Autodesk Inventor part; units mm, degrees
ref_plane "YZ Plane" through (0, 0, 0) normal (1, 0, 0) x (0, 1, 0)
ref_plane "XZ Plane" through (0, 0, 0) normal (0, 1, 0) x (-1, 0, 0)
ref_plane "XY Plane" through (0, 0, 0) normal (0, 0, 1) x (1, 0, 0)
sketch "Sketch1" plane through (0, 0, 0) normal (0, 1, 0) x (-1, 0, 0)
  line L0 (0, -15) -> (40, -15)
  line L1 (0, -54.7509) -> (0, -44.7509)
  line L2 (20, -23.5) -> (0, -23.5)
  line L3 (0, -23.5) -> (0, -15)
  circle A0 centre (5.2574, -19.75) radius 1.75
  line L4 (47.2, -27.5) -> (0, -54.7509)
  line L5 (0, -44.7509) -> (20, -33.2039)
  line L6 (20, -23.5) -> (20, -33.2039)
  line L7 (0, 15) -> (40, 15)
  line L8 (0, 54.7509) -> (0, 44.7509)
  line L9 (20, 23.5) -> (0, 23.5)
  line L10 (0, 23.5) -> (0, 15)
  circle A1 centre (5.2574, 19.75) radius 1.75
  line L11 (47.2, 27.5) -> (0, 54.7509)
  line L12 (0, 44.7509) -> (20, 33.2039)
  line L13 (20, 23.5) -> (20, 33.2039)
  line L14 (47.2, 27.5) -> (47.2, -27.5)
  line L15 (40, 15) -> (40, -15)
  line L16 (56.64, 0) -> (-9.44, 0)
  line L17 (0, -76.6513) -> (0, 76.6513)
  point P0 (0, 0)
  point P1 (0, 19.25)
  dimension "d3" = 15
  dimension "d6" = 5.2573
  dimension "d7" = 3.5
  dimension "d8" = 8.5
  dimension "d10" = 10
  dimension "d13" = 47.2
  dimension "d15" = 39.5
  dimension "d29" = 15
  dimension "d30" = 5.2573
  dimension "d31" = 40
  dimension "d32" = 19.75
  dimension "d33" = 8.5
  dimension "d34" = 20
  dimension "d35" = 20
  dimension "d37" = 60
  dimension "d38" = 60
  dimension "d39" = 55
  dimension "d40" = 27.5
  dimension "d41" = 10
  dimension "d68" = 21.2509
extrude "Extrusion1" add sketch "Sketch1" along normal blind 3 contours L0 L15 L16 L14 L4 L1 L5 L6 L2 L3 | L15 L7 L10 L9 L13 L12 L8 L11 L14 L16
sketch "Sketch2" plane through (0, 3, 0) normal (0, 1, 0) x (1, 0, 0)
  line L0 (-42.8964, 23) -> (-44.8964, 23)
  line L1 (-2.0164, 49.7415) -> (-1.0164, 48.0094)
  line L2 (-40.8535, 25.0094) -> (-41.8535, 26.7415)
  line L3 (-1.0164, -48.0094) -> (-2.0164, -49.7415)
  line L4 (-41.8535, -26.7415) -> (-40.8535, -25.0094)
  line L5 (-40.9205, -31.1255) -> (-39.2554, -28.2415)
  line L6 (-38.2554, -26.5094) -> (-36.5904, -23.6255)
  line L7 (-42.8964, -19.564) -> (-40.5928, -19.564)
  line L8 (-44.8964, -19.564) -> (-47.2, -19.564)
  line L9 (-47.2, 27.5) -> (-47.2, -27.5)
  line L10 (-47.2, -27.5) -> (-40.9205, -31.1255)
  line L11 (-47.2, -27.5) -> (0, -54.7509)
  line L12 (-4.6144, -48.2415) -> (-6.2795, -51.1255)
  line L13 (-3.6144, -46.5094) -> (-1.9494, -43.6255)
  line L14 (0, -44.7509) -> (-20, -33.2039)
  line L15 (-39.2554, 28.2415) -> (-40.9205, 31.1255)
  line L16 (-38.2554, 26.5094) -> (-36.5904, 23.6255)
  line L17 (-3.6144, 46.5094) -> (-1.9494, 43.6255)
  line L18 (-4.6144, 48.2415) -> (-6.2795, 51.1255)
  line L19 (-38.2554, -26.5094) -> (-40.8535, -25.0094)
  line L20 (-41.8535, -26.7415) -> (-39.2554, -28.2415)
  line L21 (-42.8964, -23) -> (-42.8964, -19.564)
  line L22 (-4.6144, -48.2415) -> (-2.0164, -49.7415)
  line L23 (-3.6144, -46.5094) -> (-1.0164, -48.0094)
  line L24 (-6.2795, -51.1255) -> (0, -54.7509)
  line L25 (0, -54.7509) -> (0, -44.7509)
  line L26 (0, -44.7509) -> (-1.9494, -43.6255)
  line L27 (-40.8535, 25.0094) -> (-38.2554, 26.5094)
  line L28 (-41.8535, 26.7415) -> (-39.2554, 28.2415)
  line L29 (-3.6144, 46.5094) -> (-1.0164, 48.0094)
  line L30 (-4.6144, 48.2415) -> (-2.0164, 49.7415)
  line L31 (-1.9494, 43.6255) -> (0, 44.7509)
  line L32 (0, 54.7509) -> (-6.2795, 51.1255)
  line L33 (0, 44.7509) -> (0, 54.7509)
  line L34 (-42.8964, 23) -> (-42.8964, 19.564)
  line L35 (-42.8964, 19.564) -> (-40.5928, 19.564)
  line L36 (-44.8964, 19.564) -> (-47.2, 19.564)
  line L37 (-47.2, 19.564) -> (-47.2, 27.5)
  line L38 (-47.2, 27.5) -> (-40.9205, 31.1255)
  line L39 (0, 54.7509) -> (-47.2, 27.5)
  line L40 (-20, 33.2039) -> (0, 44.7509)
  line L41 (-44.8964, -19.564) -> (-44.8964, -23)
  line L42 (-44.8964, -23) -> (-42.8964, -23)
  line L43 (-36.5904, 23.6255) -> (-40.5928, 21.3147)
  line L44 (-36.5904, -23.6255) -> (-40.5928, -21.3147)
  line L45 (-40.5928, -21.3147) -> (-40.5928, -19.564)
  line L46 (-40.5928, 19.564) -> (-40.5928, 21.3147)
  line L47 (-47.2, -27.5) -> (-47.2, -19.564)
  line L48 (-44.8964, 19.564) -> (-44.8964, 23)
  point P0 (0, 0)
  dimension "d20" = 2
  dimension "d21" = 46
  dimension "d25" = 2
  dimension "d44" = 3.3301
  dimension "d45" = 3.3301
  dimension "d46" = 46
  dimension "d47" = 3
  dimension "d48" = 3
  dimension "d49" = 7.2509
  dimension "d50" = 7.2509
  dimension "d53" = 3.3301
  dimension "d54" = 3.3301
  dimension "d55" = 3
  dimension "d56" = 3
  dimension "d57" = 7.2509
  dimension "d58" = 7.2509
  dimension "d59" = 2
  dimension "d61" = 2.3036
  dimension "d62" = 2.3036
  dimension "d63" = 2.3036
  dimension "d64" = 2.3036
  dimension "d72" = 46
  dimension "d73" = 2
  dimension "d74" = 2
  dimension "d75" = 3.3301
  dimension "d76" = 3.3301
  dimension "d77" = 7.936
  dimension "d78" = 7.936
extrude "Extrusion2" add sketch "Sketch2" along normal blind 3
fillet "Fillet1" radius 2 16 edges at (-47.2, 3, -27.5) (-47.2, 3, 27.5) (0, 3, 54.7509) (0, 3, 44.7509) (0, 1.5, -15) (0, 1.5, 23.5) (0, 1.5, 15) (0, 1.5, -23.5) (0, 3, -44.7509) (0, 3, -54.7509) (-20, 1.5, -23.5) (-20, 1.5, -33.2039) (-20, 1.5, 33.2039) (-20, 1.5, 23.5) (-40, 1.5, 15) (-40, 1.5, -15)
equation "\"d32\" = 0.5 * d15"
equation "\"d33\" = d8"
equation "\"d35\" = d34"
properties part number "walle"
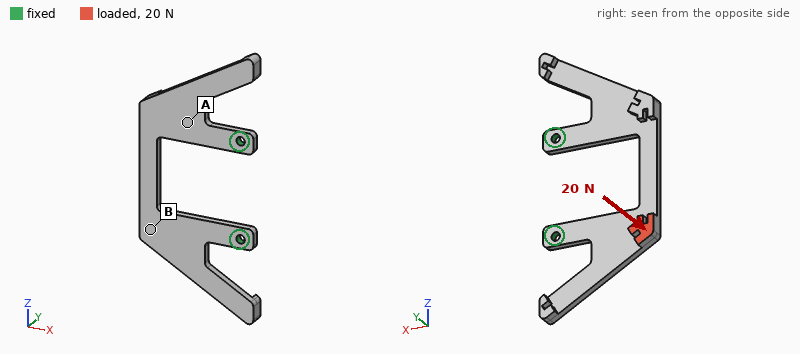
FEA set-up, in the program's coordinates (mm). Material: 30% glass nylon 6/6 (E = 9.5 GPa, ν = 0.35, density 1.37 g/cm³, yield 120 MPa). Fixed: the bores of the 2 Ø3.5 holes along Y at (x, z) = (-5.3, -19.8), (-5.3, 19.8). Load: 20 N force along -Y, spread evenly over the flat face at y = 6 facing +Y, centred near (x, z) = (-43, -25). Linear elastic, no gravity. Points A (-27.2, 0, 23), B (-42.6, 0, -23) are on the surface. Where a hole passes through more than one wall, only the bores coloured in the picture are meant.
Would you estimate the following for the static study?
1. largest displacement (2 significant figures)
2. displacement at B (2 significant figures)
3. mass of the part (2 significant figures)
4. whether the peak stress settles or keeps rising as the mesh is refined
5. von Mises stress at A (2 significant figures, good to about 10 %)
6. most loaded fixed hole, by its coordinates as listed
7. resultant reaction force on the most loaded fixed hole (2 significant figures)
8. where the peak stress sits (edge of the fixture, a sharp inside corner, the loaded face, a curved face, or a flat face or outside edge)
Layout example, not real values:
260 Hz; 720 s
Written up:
1.4 mm; 1.1 mm; 9.2 g; keeps rising; 6.1 MPa; (-5.3, -19.8); 17 N; edge of the fixture
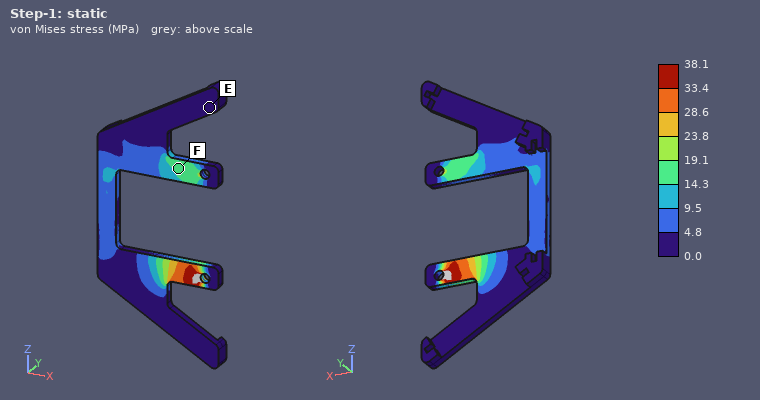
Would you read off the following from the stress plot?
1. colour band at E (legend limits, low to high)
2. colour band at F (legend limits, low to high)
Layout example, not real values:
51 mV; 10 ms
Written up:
0.0 to 4.8 MPa; 14.3 to 19.1 MPa
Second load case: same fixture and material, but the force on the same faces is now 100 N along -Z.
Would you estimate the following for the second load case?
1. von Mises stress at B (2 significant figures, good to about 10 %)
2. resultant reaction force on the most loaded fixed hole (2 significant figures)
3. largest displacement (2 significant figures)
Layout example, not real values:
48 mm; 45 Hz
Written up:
11 MPa; 71 N; 0.66 mm
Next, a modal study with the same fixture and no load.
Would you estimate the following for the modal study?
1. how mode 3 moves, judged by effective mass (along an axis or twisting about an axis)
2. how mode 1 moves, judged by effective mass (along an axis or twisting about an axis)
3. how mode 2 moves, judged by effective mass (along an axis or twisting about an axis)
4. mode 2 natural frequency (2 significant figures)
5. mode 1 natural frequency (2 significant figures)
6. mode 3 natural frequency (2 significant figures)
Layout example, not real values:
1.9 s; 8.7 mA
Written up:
along Y; along Y; twisting about X; 540 Hz; 410 Hz; 590 Hz
